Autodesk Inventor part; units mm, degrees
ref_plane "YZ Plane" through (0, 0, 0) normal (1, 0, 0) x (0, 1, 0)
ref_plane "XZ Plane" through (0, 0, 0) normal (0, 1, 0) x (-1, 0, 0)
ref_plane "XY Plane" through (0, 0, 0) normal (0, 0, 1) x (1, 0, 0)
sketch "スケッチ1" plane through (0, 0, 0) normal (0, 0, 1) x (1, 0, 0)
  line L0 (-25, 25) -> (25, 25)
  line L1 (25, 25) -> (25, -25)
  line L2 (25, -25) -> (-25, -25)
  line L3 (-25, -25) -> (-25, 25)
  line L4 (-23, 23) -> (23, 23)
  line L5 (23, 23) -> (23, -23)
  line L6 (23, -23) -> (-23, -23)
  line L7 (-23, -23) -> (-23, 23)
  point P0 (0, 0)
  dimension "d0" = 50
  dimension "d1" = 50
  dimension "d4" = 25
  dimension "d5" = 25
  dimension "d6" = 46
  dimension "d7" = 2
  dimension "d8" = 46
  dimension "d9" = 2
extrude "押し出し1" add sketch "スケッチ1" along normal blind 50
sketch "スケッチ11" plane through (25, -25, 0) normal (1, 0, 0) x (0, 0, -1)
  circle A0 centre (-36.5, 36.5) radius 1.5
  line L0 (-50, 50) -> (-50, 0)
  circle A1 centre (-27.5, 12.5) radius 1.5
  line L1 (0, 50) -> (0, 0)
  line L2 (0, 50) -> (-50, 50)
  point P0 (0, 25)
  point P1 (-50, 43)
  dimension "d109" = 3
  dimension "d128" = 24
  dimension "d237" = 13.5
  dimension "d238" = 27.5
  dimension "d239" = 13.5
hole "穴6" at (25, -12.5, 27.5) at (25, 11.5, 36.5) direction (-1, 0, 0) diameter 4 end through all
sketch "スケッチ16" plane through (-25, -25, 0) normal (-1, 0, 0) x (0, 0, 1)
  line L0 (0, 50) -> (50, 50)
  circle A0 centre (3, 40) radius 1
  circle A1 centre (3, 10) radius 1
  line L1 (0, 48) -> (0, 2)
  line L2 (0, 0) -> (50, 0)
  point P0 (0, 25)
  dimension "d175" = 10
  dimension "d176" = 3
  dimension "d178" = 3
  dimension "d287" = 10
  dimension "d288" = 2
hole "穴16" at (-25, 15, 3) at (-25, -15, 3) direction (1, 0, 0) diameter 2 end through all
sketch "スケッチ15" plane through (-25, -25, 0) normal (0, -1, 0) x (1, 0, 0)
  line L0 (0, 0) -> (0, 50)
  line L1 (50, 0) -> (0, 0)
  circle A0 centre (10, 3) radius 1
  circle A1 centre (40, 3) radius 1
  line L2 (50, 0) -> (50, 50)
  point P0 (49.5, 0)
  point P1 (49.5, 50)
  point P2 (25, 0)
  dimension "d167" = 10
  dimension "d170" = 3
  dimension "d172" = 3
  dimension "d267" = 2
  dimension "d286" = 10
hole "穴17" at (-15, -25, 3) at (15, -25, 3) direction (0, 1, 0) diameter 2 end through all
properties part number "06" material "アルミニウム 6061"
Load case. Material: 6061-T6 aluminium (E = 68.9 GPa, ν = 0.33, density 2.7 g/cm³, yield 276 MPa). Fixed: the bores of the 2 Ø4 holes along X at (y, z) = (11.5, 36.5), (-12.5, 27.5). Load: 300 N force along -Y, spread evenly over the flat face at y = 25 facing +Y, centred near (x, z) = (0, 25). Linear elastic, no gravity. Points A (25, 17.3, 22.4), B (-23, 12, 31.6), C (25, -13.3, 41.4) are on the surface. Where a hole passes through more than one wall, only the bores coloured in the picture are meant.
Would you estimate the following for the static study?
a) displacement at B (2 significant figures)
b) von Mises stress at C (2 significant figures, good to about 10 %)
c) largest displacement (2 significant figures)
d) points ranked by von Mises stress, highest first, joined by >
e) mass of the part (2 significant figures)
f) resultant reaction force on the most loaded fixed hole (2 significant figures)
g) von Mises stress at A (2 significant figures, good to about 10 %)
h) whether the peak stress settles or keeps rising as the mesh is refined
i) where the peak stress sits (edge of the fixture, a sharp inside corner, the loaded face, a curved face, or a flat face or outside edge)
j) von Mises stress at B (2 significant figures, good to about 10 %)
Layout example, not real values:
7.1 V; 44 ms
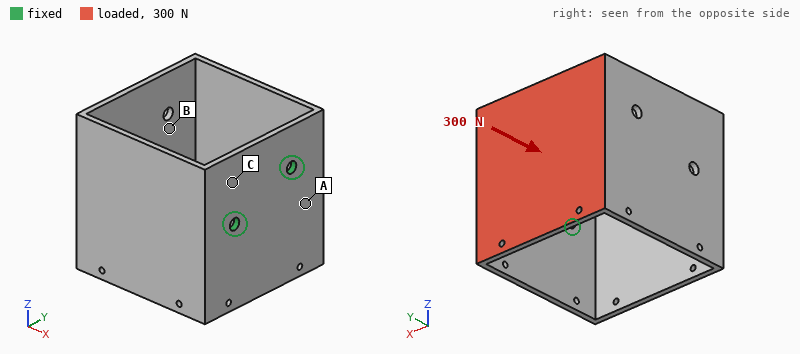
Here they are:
0.86 mm; 46 MPa; 0.91 mm; A > C > B; 51 g; 230 N; 63 MPa; keeps rising; edge of the fixture; 15 MPa
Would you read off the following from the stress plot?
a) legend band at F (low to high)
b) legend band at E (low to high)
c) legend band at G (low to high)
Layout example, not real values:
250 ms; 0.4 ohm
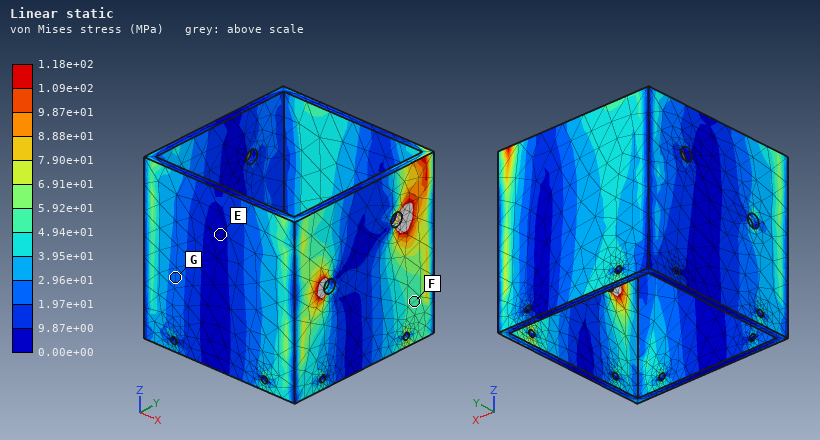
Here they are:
4.94e+01 to 5.92e+01 MPa; 0.00e+00 to 9.87e+00 MPa; 1.97e+01 to 2.96e+01 MPa
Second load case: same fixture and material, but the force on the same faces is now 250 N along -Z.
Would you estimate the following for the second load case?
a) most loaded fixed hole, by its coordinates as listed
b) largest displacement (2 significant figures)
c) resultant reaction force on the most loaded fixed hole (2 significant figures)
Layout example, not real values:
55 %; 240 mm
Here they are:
(11.5, 36.5); 0.81 mm; 350 N
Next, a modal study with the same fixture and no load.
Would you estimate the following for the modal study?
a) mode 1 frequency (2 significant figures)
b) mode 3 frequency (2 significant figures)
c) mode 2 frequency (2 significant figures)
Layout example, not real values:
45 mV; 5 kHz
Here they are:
430 Hz; 1100 Hz; 520 Hz
